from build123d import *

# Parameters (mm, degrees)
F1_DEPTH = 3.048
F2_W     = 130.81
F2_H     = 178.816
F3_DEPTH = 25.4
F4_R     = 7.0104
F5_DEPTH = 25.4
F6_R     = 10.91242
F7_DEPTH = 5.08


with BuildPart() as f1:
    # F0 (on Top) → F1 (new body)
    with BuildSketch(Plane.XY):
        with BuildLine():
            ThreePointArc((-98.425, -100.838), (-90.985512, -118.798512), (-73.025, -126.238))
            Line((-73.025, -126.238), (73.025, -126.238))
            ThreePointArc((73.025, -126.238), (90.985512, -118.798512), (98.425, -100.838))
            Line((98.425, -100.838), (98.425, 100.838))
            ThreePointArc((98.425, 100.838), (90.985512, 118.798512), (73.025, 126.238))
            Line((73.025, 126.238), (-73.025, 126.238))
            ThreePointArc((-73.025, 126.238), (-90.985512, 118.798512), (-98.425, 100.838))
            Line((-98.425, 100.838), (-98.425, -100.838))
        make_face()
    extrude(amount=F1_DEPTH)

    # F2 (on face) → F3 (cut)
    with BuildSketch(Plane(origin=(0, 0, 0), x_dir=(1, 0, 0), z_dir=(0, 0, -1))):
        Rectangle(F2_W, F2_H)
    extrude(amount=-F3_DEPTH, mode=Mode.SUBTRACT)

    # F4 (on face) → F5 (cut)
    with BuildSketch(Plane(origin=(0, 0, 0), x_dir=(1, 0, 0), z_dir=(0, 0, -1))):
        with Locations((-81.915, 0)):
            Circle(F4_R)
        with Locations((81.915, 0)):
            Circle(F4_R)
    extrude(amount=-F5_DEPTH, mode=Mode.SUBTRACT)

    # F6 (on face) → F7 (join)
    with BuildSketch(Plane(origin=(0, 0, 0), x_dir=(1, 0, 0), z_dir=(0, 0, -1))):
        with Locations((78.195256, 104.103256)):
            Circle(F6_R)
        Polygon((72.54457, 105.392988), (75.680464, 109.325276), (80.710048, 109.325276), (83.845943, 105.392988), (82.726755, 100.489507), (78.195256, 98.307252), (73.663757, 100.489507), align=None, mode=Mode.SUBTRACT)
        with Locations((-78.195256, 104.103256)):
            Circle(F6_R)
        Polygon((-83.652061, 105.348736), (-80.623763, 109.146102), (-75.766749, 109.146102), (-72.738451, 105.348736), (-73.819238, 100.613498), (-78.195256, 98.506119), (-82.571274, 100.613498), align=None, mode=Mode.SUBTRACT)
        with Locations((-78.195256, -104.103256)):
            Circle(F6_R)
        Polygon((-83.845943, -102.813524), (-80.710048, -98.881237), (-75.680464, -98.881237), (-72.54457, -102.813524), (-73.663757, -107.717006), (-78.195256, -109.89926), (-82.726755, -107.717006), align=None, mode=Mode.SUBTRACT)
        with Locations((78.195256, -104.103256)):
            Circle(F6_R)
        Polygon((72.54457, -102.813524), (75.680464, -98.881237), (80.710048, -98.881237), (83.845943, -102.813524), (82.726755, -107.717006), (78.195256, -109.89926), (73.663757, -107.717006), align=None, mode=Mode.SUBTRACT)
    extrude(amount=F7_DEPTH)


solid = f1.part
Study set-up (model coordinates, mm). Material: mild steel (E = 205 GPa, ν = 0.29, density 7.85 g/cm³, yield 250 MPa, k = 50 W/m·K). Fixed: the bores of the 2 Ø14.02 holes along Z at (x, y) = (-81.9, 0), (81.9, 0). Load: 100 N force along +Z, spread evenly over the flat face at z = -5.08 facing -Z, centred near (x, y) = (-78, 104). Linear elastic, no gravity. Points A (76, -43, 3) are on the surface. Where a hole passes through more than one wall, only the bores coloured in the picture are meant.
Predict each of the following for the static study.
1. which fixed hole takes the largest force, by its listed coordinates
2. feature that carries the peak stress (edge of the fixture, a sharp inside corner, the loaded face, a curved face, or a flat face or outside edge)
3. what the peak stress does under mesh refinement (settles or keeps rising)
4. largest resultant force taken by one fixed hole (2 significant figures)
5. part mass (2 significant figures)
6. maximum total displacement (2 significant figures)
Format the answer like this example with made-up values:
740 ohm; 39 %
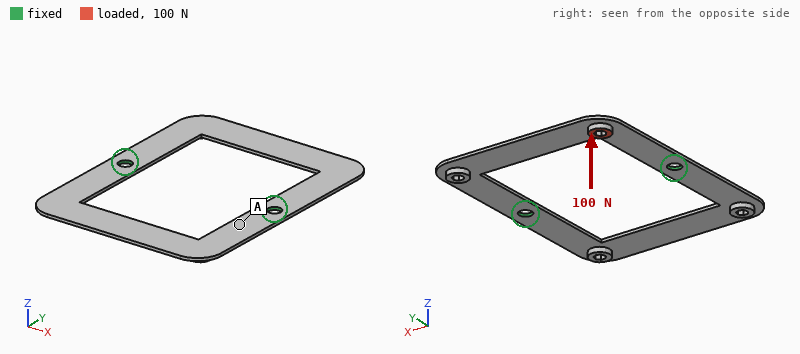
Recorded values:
(-81.9, 0); edge of the fixture; keeps rising; 88 N; 650 g; 1.7 mm
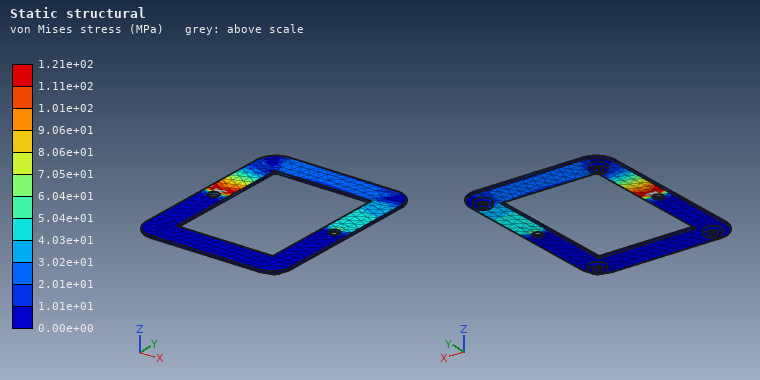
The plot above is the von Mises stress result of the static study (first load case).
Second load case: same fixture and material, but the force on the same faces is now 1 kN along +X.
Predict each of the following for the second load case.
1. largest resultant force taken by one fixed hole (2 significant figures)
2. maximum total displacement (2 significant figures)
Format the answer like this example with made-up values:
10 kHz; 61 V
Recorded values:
610 N; 0.42 mm
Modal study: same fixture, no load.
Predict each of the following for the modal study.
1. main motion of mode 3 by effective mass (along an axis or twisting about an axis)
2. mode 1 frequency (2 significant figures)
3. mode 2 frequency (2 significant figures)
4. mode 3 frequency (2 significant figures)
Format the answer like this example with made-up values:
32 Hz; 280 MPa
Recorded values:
twisting about Y; 100 Hz; 100 Hz; 240 Hz
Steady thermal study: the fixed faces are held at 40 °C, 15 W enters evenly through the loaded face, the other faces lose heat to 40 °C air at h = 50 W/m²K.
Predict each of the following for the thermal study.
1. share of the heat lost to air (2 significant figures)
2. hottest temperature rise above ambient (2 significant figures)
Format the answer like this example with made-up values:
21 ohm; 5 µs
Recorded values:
94 %; 51 K
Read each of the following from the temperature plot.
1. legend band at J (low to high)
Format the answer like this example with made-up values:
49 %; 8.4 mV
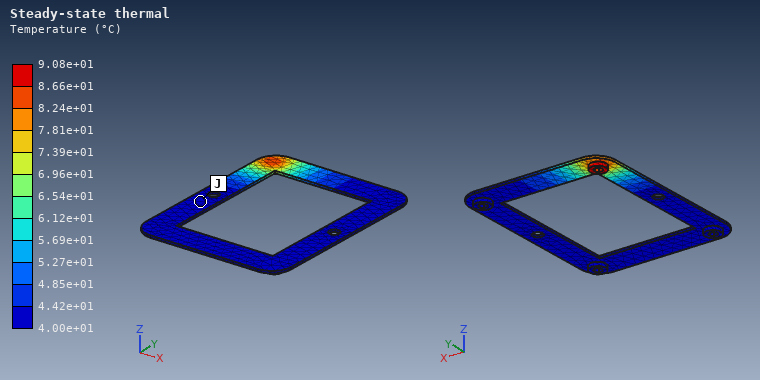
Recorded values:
4.00e+01 to 4.42e+01 °C
